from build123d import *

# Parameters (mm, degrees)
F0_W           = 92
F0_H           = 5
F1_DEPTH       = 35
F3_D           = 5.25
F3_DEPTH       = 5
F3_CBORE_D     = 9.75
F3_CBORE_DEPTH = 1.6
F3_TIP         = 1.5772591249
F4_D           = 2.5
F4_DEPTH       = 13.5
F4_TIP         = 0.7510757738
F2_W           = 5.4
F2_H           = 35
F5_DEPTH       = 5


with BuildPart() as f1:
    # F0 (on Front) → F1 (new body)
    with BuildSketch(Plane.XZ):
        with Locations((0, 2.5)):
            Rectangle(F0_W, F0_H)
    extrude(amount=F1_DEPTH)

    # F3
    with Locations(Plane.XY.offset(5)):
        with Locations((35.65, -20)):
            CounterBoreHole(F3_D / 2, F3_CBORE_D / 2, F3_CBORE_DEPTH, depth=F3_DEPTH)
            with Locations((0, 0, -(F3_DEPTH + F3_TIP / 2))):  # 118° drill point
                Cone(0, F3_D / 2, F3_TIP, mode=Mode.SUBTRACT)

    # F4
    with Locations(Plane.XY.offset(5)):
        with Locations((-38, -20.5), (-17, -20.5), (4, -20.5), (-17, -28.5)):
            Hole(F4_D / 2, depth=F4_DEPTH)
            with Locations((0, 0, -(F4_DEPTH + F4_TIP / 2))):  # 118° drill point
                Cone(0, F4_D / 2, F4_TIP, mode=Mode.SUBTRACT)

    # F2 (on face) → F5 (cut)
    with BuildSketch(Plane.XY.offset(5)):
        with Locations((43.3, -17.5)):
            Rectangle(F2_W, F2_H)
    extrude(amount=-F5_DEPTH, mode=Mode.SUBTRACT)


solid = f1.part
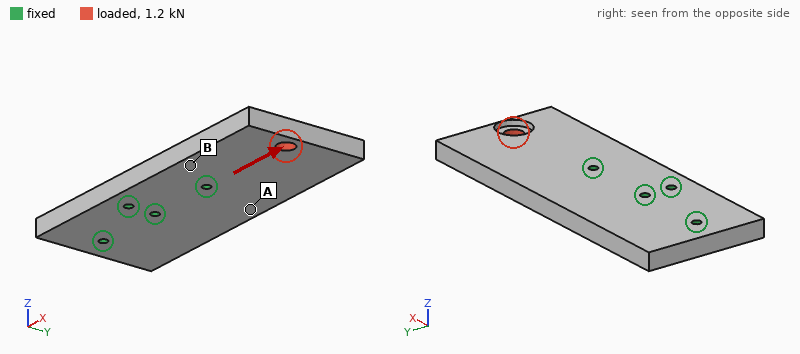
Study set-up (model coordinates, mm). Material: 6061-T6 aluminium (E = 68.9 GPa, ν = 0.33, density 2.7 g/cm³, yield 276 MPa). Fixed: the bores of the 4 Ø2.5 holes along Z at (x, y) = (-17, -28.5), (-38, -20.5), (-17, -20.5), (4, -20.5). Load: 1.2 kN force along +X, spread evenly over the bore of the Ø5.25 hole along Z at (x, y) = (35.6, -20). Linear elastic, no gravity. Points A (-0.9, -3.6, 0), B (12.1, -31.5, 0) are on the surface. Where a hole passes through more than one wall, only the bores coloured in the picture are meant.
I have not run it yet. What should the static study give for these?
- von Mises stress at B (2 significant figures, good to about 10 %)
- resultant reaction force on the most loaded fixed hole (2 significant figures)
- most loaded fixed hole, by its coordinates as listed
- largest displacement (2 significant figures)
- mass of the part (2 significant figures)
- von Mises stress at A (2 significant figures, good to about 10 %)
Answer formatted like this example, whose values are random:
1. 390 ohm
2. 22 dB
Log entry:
1. 13 MPa
2. 760 N
3. (4, -20.5)
4. 33 µm
5. 40 g
6. 5.8 MPa
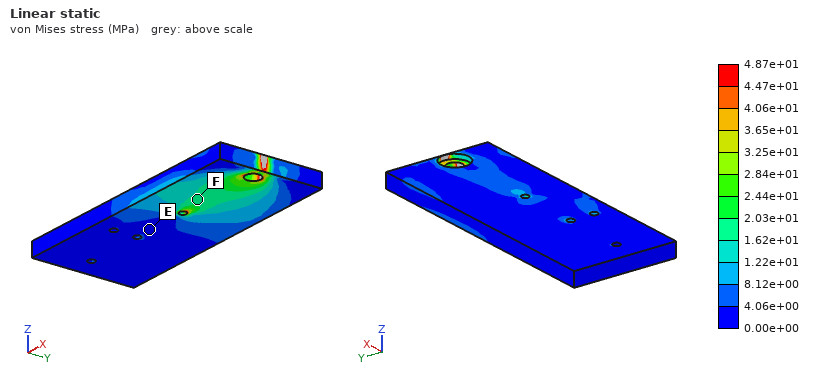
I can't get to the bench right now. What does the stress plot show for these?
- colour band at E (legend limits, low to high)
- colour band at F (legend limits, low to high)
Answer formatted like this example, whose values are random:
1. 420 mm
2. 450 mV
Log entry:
1. 0.00e+00 to 4.06e+00 MPa
2. 1.62e+01 to 2.03e+01 MPa
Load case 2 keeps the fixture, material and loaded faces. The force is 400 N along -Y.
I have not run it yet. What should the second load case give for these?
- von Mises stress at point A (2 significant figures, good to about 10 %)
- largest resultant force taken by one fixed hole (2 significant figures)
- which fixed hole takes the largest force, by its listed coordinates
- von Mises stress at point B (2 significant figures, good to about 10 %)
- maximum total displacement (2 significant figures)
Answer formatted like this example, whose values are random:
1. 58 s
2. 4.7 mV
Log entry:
1. 7.9 MPa
2. 740 N
3. (4, -20.5)
4. 8.4 MPa
5. 19 µm
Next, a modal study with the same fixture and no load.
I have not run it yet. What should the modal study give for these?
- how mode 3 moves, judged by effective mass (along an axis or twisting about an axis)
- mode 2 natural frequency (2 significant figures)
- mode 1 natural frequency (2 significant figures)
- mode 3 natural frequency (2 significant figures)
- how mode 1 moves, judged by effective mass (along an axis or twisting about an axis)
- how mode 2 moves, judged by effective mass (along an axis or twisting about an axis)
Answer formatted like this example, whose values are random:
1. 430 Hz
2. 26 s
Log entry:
1. along Z
2. 4900 Hz
3. 2700 Hz
4. 8700 Hz
5. along Z
6. twisting about X
